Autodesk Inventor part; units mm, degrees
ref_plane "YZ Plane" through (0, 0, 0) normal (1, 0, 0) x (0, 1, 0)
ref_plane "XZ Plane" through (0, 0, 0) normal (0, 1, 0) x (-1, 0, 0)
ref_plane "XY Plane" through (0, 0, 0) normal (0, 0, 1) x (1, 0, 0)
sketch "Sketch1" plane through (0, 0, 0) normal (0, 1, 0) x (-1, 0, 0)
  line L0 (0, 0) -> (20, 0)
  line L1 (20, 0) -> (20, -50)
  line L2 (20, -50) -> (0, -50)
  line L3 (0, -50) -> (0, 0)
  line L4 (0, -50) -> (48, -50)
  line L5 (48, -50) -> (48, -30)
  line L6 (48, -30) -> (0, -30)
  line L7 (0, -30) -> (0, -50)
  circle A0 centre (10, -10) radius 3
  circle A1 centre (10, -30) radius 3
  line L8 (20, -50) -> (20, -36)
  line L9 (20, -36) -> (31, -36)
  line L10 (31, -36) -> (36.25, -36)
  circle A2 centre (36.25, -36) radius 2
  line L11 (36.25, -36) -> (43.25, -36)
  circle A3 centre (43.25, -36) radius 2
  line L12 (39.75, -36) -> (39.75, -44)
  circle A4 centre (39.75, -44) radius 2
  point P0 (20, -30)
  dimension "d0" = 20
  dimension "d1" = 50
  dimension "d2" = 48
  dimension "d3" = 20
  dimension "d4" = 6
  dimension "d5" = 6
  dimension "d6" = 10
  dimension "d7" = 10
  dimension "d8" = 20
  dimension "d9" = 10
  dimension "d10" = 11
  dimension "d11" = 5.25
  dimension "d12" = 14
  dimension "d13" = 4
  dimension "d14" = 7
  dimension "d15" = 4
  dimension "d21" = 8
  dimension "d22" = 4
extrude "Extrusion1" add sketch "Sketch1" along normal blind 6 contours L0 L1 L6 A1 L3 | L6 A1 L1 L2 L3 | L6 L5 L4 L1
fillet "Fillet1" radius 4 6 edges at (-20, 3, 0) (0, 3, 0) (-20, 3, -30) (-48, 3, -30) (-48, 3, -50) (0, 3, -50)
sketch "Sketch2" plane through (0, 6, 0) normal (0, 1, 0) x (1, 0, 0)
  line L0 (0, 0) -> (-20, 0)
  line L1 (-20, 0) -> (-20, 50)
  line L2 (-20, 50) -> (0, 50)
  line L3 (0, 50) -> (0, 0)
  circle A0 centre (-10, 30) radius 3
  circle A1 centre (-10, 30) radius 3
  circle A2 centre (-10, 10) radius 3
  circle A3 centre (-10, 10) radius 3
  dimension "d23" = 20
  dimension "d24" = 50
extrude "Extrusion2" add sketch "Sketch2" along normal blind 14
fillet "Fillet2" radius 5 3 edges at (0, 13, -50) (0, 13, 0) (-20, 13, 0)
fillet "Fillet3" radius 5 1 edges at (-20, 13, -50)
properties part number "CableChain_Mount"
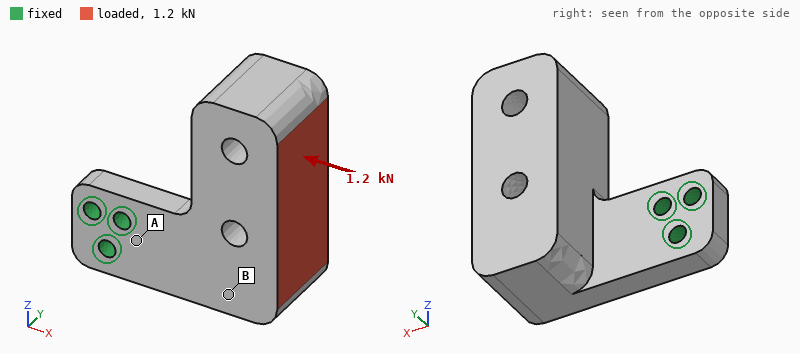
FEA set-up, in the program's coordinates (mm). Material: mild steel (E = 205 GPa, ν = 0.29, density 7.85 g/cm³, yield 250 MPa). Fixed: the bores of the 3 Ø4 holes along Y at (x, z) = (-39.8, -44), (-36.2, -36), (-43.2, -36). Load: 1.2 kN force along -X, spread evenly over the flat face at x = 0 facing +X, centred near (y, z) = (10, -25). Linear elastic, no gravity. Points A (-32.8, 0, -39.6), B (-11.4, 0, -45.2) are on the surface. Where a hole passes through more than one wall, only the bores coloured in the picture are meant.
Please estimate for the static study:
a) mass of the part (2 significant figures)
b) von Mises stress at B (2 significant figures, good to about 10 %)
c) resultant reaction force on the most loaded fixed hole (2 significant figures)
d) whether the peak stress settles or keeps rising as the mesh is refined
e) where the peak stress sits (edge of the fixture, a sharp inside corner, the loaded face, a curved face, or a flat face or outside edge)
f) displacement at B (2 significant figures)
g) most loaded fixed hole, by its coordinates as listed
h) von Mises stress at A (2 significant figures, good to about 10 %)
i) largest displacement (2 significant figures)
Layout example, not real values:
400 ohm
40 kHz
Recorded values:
170 g
17 MPa
1.9 kN
keeps rising
edge of the fixture
35 µm
(-36.2, -36)
56 MPa
83 µm
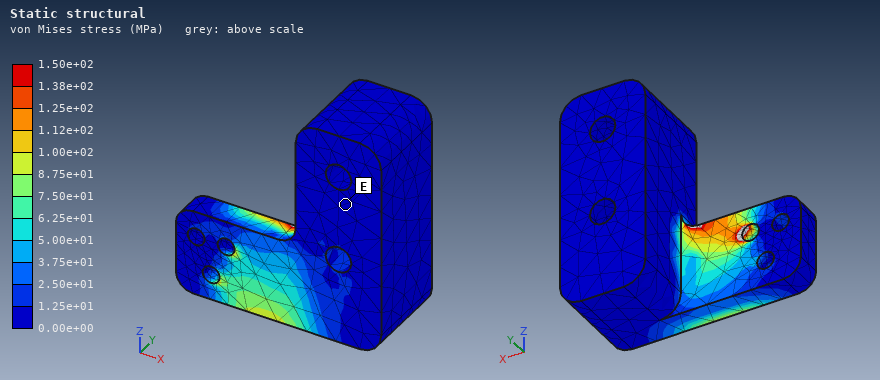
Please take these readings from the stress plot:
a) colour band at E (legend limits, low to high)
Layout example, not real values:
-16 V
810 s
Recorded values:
0.00e+00 to 1.25e+01 MPa
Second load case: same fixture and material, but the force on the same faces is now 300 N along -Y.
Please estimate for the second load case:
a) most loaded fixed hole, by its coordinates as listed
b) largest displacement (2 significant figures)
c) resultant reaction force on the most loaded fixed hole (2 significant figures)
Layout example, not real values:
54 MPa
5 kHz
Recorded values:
(-36.2, -36)
85 µm
740 N
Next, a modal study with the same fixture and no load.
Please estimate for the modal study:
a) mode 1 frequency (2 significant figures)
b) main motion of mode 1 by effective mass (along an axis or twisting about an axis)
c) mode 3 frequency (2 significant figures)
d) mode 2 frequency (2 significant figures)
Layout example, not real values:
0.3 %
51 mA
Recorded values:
1100 Hz
along Y
3000 Hz
2000 Hz
